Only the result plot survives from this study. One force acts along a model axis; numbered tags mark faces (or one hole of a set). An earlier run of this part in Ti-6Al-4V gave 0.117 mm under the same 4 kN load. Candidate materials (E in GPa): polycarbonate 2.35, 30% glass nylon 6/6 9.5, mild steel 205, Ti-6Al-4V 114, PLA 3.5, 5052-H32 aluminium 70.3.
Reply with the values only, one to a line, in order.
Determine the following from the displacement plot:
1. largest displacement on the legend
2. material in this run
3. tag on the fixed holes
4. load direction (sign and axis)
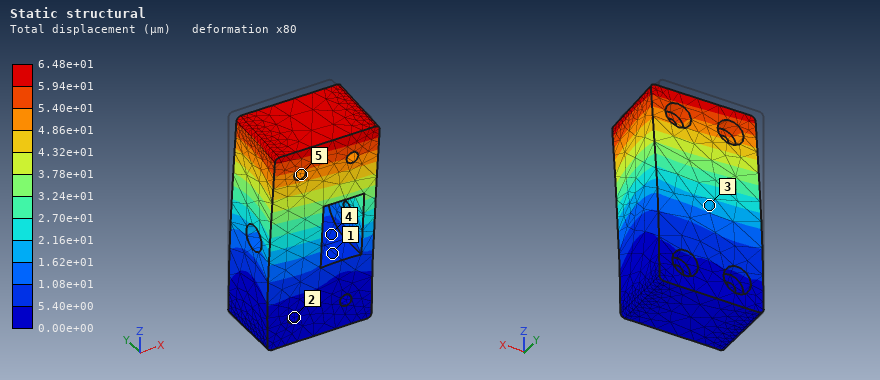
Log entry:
6.48e+01 µm
mild steel
2
-Y
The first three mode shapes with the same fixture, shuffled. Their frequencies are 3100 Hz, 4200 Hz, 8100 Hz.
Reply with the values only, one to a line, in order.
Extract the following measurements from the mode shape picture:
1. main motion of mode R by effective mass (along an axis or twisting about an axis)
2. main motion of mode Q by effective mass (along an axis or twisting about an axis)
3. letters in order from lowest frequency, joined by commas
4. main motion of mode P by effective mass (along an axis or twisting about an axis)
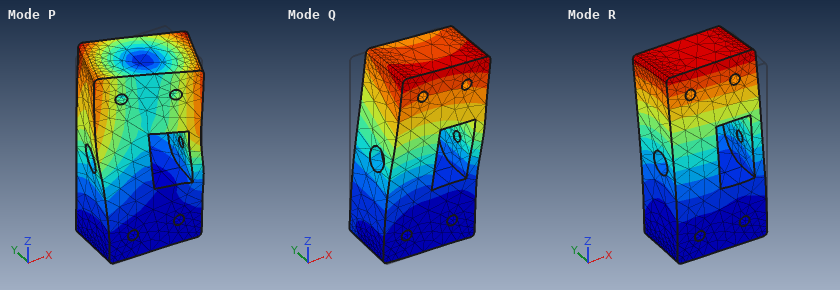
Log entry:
along Y
along X
R, Q, P
twisting about Z
